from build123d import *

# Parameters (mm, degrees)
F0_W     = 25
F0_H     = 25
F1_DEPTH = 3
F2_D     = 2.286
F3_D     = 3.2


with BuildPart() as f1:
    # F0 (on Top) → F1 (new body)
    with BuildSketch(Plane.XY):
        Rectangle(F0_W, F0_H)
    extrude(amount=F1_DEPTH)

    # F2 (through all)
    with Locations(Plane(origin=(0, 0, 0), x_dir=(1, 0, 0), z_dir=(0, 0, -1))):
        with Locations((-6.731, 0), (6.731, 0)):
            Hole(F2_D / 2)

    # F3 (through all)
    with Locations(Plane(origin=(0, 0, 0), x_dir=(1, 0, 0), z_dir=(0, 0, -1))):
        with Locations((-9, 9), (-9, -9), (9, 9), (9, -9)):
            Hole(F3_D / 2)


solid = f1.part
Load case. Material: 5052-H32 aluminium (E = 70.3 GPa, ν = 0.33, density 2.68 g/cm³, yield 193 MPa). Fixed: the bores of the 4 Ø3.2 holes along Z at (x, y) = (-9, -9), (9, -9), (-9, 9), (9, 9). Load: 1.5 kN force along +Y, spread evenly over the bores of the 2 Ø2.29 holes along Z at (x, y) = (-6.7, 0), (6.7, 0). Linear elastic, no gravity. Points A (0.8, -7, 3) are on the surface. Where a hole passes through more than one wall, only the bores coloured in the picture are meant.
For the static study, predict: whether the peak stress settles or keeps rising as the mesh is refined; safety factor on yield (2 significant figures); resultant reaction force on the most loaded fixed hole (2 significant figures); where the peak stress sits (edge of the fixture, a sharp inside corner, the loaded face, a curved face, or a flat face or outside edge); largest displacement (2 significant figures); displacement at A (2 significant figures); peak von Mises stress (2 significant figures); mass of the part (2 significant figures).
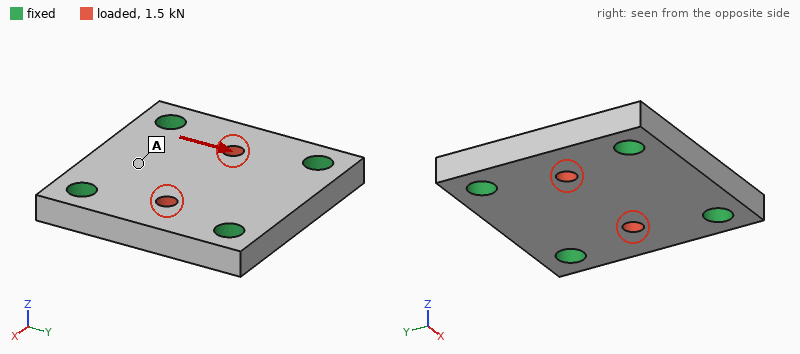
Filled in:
settles
3.2
390 N
the loaded face
2.7 µm
1.4 µm
61 MPa
4.7 g
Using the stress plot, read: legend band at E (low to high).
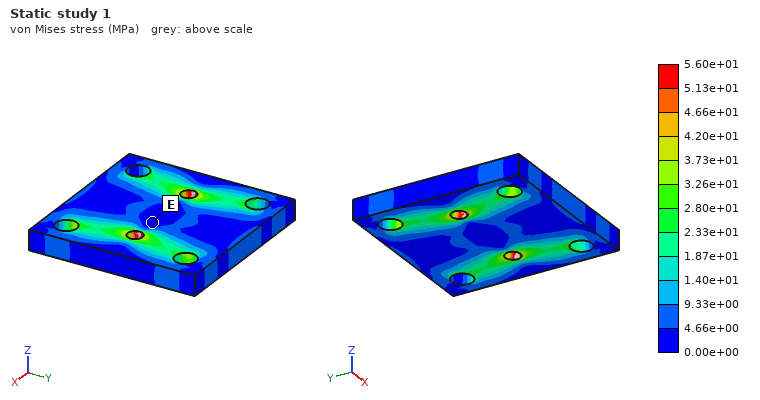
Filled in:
0.00e+00 to 4.66e+00 MPa
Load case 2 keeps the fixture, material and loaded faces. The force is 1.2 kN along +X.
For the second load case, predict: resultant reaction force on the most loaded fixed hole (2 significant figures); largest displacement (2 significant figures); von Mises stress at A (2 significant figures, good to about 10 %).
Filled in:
320 N
3.7 µm
12 MPa
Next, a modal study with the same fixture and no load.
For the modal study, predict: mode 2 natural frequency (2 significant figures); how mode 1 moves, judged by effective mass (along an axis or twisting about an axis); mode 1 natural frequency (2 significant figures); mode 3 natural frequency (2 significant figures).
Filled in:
53 kHz
along Z
36 kHz
53 kHz
